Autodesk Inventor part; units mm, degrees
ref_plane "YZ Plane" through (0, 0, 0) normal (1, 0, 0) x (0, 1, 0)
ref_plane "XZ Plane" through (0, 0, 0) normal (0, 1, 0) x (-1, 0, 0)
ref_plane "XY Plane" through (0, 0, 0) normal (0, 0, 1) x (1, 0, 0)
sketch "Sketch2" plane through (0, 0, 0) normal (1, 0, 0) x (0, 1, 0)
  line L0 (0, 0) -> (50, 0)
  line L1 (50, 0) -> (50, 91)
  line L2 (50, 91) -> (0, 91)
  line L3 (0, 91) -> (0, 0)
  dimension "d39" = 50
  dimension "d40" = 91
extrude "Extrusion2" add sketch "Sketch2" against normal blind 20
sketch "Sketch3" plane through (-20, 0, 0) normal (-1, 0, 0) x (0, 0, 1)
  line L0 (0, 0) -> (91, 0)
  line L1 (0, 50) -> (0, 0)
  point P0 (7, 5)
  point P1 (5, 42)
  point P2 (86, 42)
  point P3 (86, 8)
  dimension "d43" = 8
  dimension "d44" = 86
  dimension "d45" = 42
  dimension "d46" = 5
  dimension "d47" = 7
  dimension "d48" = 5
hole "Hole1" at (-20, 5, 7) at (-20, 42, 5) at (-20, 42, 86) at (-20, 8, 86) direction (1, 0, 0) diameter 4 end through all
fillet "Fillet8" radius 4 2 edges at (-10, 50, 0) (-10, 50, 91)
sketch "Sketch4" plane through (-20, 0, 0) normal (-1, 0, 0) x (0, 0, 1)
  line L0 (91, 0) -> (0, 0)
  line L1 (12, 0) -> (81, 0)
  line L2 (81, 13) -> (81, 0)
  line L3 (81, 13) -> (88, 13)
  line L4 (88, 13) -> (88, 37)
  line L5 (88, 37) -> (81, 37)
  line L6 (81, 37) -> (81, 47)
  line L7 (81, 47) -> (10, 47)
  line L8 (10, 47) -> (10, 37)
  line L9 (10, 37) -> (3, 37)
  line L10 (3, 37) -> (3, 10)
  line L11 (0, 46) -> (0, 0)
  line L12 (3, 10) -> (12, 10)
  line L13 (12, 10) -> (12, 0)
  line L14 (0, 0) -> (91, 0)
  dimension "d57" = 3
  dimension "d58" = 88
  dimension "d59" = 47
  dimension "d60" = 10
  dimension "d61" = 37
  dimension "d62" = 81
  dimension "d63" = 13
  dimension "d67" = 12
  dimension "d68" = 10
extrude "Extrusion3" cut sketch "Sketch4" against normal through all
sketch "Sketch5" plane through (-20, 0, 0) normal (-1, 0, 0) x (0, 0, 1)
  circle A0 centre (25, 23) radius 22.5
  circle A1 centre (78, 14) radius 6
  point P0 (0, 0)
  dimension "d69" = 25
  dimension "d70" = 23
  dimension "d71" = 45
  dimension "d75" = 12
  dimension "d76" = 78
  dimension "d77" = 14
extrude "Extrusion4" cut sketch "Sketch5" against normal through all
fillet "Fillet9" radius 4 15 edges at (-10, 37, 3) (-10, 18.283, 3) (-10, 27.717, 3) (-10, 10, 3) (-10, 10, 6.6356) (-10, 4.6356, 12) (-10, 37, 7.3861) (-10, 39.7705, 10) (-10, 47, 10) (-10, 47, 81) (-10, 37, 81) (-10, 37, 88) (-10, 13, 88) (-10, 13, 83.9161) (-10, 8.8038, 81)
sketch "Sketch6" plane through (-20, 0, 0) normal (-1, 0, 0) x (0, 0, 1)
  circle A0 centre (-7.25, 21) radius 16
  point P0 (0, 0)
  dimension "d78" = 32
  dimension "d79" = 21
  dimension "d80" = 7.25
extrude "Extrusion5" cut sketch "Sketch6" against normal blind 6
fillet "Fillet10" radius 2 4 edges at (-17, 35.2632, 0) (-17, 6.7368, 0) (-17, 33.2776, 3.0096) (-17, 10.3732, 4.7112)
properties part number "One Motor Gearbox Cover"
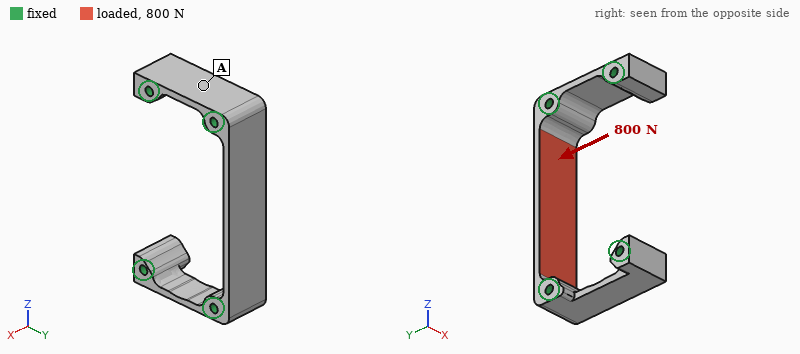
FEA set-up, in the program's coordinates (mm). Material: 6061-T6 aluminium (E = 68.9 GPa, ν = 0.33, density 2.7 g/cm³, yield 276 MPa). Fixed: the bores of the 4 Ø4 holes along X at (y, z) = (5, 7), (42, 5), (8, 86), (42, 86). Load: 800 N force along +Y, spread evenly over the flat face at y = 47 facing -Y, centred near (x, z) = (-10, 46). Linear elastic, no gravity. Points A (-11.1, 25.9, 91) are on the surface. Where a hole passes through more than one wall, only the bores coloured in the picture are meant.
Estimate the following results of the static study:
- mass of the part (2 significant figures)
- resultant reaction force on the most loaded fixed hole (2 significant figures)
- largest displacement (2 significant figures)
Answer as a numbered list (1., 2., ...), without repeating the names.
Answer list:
1. 42 g
2. 590 N
3. 0.26 mm
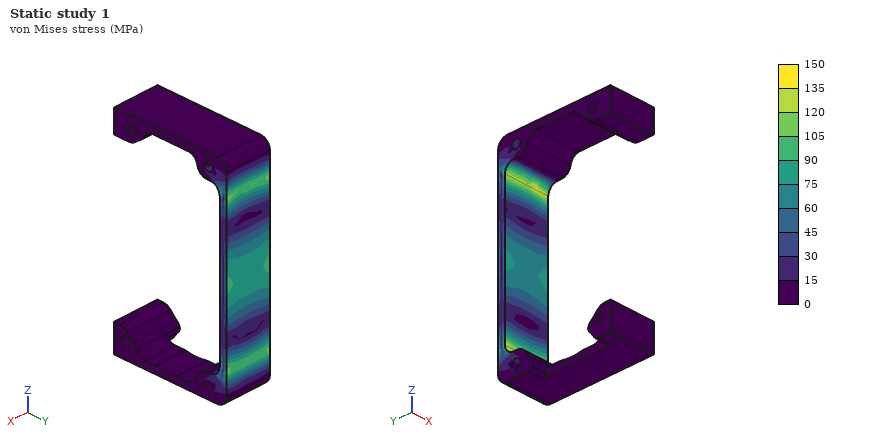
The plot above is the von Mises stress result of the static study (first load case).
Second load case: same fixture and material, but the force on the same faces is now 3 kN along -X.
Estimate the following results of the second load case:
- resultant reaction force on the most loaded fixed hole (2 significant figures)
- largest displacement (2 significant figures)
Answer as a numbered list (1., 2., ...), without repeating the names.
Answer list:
1. 1.5 kN
2. 0.12 mm
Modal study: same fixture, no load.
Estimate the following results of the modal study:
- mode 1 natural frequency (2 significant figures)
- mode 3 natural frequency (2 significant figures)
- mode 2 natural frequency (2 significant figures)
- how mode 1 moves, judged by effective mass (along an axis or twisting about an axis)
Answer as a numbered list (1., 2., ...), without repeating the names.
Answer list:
1. 3200 Hz
2. 8500 Hz
3. 7300 Hz
4. along Y
